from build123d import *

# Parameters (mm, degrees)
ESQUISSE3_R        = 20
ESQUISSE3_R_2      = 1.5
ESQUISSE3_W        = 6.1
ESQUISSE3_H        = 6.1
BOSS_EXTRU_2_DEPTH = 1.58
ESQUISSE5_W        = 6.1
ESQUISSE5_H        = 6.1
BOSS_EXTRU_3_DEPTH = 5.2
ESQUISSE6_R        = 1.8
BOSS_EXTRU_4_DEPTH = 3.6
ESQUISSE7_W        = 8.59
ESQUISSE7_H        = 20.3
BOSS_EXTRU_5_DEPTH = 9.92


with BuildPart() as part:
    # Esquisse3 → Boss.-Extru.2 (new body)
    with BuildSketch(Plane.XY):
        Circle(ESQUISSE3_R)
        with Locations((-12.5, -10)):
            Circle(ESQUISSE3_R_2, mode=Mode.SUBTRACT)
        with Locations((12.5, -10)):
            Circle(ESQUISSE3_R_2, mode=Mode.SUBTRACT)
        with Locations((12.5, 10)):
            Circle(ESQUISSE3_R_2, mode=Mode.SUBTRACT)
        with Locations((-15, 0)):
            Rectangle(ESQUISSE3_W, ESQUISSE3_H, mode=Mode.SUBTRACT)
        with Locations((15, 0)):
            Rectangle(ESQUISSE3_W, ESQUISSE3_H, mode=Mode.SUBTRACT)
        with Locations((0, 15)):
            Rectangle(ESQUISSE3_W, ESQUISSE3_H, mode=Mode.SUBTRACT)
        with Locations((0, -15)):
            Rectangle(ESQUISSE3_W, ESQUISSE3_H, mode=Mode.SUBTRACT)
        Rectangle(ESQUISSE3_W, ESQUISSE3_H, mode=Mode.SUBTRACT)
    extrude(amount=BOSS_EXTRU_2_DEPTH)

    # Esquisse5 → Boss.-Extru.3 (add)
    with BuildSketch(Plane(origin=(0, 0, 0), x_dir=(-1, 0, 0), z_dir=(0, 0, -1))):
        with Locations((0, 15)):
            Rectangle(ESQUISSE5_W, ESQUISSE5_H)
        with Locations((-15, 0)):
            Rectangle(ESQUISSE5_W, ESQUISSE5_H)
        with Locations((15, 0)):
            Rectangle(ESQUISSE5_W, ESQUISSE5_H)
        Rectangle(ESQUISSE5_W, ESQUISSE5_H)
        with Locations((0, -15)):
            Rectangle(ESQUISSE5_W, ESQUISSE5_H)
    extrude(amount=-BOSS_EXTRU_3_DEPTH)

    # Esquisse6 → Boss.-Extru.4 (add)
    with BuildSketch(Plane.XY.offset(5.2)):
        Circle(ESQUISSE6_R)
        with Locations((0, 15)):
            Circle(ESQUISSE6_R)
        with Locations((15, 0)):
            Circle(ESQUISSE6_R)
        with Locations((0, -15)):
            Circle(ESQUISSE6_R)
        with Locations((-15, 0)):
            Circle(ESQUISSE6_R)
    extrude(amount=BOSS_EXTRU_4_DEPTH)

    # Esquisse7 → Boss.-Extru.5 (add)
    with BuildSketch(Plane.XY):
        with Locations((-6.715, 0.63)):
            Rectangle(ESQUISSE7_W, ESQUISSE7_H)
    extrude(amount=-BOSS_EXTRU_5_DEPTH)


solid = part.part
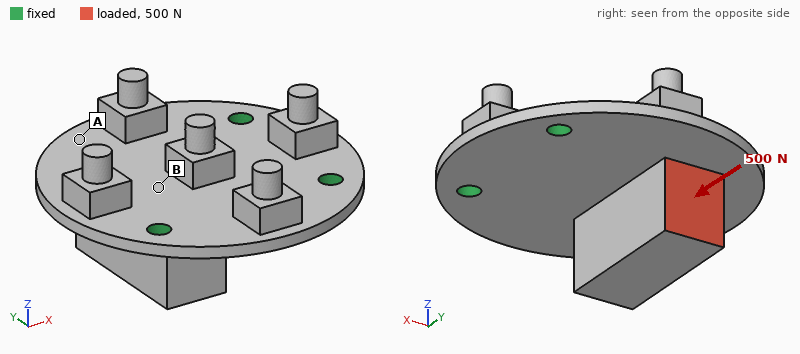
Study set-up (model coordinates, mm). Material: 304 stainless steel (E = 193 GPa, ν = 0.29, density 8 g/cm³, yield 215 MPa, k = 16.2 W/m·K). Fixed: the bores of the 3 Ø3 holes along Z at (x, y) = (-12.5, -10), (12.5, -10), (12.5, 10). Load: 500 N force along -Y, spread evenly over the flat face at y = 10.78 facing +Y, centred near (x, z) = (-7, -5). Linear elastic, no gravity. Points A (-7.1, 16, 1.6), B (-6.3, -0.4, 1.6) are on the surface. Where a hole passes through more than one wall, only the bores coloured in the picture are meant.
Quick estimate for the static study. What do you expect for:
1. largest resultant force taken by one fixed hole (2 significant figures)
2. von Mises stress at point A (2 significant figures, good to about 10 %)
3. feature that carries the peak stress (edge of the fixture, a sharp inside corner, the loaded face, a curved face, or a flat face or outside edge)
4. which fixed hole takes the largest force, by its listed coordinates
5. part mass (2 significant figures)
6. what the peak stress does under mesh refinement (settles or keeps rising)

360 N
37 MPa
edge of the fixture
(-12.5, -10)
36 g
keeps rising
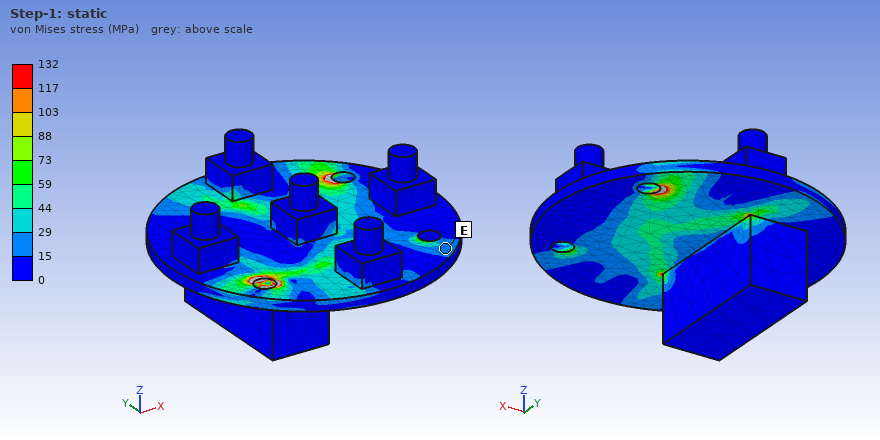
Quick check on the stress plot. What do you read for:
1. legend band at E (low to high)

15 to 29 MPa
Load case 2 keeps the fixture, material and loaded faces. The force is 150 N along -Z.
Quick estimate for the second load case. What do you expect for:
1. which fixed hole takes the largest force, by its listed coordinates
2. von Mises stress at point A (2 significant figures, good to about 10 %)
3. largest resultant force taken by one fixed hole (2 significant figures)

(12.5, 10)
37 MPa
100 N
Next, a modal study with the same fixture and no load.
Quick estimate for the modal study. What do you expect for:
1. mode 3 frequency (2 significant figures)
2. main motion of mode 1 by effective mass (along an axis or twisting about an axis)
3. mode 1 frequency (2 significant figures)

9200 Hz
along Z
3100 Hz
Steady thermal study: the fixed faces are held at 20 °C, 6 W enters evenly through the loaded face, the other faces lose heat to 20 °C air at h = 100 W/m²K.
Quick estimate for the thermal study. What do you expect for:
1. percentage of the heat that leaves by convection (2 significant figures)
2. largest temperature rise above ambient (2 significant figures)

75 %
53 K
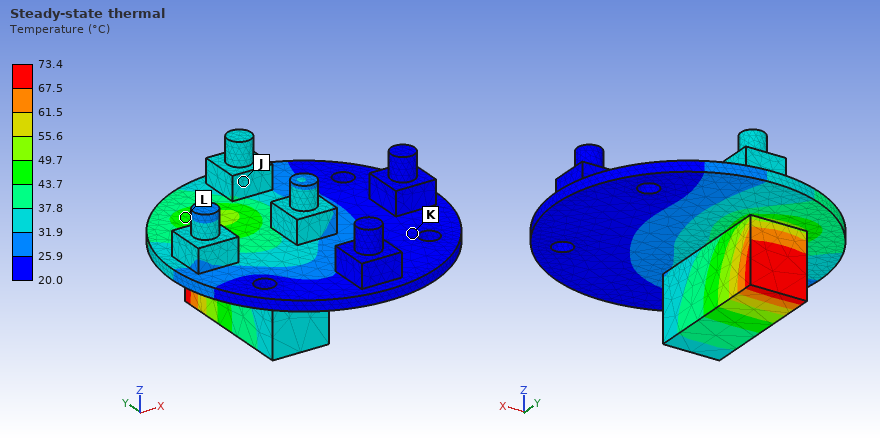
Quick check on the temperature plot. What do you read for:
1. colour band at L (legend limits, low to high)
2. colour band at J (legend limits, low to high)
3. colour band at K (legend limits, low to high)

43.7 to 49.7 °C
31.9 to 37.8 °C
20.0 to 25.9 °C
